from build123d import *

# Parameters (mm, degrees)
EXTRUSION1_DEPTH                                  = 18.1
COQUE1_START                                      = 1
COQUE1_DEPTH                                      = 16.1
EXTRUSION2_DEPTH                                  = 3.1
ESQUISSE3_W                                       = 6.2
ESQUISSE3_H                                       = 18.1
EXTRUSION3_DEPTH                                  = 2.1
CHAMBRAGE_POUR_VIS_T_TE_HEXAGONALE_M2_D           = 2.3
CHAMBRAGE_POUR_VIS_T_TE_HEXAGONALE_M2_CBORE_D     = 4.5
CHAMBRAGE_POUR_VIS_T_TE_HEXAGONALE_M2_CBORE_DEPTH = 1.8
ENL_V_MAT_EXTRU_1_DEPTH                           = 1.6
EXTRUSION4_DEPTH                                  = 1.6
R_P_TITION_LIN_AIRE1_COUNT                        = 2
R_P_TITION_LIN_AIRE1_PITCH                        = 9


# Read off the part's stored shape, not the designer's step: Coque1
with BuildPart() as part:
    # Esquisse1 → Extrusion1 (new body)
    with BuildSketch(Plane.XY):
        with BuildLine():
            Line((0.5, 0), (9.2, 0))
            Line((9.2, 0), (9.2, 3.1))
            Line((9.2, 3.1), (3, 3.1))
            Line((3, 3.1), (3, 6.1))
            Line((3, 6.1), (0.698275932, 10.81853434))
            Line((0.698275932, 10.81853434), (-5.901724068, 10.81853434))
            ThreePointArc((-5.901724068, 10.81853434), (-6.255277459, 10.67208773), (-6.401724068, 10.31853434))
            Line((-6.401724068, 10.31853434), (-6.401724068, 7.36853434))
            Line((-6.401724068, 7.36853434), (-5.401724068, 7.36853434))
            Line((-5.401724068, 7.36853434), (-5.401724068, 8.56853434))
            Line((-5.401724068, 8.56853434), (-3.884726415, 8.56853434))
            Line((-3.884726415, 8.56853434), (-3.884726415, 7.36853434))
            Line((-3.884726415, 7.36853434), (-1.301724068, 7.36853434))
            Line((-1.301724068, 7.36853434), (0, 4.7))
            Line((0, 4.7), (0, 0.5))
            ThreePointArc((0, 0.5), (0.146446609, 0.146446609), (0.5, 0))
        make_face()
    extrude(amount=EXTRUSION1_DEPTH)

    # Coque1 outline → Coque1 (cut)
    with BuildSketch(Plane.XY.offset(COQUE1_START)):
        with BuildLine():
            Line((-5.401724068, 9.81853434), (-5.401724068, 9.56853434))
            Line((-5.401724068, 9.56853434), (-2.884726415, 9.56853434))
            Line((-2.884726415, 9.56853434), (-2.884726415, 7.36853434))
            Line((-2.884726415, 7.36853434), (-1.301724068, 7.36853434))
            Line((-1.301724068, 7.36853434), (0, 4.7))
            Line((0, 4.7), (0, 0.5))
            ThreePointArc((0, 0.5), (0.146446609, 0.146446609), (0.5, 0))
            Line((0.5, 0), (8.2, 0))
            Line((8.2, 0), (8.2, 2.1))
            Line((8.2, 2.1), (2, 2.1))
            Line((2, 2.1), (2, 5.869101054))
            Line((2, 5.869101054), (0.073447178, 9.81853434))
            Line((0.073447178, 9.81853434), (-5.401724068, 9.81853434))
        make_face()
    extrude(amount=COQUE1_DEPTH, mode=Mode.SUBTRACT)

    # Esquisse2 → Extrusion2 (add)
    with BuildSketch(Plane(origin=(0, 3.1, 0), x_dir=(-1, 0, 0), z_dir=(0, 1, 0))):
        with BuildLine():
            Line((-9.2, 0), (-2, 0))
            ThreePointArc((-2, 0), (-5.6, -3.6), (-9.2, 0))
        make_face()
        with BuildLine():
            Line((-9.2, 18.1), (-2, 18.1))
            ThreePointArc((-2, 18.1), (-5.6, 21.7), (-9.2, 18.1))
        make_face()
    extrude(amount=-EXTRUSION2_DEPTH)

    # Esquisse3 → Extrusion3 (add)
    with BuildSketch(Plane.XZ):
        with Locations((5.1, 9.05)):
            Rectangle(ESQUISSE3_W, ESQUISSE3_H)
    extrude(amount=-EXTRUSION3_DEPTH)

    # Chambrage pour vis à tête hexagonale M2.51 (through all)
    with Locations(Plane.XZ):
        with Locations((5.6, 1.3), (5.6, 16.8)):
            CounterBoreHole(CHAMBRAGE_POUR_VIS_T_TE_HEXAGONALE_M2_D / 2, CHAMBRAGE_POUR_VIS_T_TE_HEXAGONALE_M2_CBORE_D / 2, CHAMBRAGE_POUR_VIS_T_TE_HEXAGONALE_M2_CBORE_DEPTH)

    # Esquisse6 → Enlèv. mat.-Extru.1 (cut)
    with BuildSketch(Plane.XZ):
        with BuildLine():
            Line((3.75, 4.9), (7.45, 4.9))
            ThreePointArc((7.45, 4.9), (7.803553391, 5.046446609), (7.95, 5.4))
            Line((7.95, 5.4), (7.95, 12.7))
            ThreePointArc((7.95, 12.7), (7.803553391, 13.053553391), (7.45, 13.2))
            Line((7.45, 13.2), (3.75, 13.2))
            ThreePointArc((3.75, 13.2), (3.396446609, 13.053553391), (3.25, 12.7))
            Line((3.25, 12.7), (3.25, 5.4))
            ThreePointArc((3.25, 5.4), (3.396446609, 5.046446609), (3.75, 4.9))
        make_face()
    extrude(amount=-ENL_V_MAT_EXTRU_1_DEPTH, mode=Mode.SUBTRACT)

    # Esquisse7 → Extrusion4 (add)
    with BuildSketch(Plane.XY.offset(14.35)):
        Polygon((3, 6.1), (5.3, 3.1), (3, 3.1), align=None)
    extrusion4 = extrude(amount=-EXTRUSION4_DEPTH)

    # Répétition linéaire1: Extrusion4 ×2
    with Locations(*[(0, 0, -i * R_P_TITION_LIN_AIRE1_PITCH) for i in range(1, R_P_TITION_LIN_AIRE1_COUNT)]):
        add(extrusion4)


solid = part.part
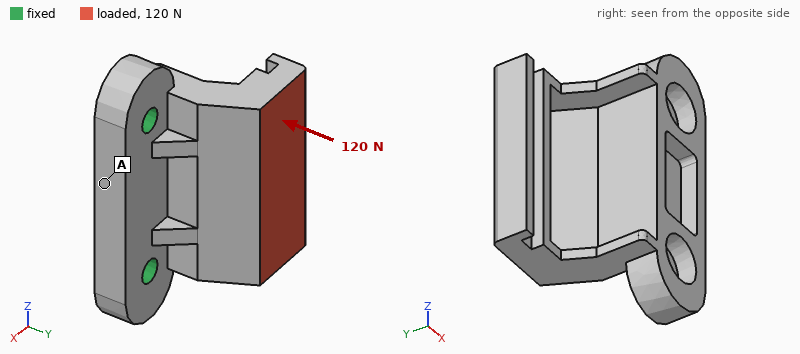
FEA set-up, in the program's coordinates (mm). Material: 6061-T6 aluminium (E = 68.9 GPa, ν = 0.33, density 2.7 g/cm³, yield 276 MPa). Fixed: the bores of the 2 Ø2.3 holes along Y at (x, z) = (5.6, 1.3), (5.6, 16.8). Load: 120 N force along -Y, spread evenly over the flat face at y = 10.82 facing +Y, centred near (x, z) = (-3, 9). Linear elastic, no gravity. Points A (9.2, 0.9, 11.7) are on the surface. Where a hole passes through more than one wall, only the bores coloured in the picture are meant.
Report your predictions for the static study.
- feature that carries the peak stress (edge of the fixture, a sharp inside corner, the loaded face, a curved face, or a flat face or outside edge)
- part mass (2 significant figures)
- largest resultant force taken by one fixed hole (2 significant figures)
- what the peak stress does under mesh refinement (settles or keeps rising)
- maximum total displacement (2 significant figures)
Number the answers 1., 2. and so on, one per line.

1. edge of the fixture
2. 2.3 g
3. 61 N
4. keeps rising
5. 97 µm
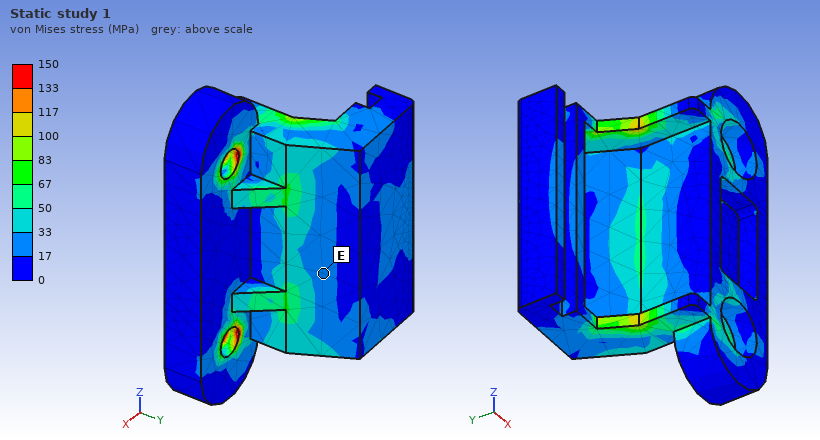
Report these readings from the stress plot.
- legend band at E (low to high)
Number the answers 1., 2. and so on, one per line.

1. 17 to 33 MPa
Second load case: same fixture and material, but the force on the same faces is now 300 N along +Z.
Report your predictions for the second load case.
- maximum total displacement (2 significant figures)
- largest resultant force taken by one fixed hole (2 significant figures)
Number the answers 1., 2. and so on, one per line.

1. 64 µm
2. 270 N
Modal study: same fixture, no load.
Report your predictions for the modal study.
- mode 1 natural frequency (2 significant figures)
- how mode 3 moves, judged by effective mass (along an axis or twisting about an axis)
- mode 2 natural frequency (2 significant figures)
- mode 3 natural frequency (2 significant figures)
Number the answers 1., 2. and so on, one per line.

1. 6000 Hz
2. along X
3. 9600 Hz
4. 21 kHz
